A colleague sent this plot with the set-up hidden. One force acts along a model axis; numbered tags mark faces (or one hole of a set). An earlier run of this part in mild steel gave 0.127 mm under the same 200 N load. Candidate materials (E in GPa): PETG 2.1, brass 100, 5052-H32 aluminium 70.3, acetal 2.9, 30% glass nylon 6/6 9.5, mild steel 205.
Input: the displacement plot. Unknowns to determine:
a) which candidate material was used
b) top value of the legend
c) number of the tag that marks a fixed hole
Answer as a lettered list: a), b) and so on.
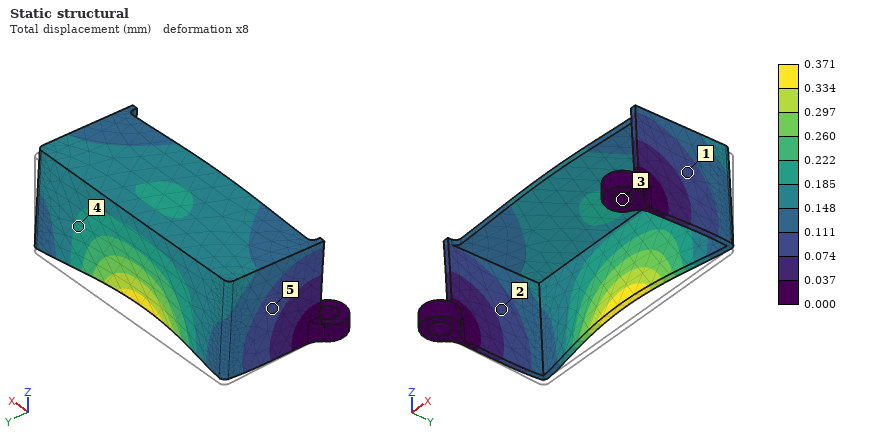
a) 5052-H32 aluminium
b) 0.371 mm
c) 3
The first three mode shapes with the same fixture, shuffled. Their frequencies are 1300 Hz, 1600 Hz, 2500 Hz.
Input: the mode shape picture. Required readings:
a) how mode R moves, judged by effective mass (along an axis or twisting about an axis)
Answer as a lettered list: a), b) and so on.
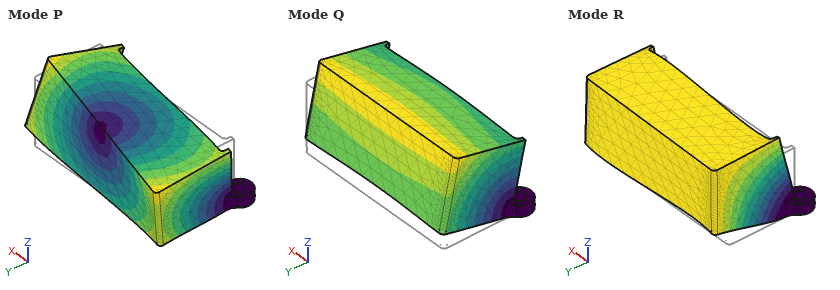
a) along X
